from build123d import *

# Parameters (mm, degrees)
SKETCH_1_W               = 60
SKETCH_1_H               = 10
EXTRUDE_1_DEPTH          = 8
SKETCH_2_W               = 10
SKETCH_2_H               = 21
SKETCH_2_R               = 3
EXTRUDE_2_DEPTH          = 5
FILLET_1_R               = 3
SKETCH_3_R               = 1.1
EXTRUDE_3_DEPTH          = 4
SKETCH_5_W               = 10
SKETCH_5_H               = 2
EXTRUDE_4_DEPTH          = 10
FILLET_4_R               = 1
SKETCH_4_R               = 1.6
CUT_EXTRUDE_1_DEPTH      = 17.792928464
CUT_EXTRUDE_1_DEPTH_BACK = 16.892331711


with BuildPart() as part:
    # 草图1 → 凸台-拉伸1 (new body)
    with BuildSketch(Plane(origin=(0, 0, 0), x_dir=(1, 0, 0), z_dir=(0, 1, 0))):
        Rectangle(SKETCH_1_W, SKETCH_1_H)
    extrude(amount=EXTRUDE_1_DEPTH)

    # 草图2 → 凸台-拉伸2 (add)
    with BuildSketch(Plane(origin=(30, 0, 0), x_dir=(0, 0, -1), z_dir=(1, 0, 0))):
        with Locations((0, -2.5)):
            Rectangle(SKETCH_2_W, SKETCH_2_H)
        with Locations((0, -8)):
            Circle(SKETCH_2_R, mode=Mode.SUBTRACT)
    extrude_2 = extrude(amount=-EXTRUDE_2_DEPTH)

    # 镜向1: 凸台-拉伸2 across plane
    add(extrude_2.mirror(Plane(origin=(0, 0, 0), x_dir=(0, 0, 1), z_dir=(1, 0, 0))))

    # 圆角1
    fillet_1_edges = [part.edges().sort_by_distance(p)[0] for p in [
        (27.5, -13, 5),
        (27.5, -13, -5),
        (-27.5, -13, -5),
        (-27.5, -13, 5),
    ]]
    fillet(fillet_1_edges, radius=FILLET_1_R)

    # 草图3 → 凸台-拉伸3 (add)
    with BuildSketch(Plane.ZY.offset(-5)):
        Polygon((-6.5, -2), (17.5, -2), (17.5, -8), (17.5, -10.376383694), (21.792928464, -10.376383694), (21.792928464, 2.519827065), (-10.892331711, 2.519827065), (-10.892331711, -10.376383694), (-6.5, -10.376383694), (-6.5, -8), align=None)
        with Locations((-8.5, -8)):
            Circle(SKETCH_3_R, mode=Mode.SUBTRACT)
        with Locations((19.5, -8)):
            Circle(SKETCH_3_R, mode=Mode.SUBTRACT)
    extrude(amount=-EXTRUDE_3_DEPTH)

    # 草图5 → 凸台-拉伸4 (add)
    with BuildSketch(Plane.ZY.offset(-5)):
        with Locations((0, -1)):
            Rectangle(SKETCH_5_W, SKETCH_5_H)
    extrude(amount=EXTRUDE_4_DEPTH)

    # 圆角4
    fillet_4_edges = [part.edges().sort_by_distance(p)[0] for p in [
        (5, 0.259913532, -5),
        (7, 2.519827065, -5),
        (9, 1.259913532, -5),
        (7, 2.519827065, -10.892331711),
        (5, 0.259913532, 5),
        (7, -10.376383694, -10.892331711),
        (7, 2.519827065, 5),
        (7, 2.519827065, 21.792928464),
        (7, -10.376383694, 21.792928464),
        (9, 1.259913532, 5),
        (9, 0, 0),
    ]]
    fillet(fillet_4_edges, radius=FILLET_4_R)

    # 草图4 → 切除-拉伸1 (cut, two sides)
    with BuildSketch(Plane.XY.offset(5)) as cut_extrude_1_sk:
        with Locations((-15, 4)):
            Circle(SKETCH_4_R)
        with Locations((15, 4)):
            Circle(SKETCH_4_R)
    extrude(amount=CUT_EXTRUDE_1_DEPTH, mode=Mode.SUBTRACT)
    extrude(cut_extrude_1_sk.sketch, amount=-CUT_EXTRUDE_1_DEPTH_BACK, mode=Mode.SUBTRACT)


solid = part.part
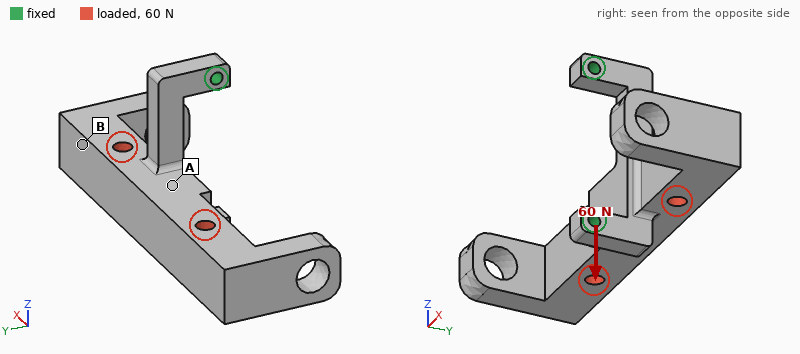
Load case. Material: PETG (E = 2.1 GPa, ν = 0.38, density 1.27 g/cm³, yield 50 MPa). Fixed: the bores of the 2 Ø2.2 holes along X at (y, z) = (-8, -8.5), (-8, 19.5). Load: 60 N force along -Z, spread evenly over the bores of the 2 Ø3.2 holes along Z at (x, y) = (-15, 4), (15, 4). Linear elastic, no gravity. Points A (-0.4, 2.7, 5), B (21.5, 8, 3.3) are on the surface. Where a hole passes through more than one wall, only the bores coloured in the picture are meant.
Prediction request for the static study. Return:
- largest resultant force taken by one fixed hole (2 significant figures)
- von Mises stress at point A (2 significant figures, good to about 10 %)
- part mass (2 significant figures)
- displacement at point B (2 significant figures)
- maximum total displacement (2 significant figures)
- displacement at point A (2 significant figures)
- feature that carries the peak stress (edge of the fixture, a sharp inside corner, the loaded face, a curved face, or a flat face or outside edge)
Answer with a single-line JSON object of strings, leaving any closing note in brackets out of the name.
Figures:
{"largest resultant force taken by one fixed hole": "39 N", "von Mises stress at point A": "2.9 MPa", "part mass": "8.3 g", "displacement at point B": "0.12 mm", "maximum total displacement": "0.73 mm", "displacement at point A": "0.22 mm", "feature that carries the peak stress": "a curved face"}
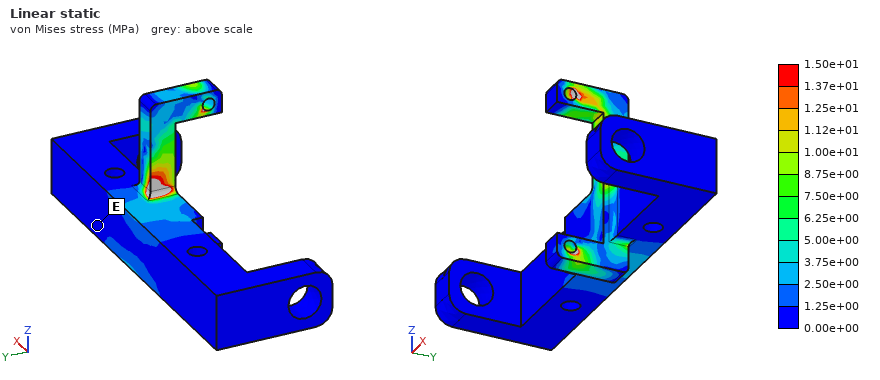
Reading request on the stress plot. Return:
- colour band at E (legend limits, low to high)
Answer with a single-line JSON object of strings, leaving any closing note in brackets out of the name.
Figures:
{"colour band at E": "0.00e+00 to 1.25e+00 MPa"}
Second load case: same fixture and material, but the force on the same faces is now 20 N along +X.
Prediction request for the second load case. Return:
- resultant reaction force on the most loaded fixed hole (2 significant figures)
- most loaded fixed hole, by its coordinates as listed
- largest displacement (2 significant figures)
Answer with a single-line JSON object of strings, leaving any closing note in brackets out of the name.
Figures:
{"resultant reaction force on the most loaded fixed hole": "14 N", "most loaded fixed hole, by its coordinates as listed": "(-8, -8.5)", "largest displacement": "0.76 mm"}
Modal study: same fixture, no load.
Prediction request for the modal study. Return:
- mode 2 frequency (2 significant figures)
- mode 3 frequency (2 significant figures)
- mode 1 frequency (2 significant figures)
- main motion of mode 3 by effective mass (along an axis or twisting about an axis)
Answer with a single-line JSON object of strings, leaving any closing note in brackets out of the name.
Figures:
{"mode 2 frequency": "470 Hz", "mode 3 frequency": "1200 Hz", "mode 1 frequency": "210 Hz", "main motion of mode 3 by effective mass": "along X"}
